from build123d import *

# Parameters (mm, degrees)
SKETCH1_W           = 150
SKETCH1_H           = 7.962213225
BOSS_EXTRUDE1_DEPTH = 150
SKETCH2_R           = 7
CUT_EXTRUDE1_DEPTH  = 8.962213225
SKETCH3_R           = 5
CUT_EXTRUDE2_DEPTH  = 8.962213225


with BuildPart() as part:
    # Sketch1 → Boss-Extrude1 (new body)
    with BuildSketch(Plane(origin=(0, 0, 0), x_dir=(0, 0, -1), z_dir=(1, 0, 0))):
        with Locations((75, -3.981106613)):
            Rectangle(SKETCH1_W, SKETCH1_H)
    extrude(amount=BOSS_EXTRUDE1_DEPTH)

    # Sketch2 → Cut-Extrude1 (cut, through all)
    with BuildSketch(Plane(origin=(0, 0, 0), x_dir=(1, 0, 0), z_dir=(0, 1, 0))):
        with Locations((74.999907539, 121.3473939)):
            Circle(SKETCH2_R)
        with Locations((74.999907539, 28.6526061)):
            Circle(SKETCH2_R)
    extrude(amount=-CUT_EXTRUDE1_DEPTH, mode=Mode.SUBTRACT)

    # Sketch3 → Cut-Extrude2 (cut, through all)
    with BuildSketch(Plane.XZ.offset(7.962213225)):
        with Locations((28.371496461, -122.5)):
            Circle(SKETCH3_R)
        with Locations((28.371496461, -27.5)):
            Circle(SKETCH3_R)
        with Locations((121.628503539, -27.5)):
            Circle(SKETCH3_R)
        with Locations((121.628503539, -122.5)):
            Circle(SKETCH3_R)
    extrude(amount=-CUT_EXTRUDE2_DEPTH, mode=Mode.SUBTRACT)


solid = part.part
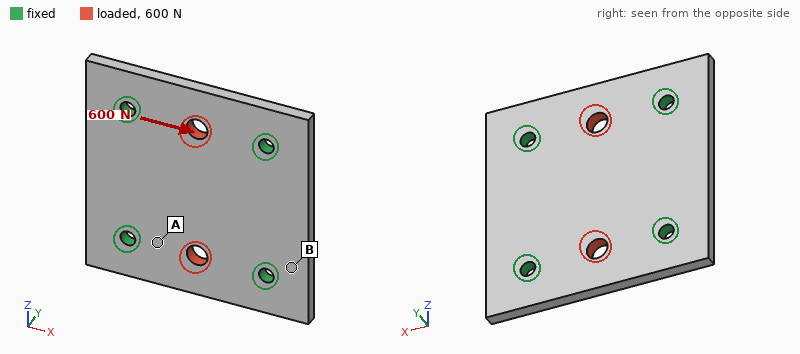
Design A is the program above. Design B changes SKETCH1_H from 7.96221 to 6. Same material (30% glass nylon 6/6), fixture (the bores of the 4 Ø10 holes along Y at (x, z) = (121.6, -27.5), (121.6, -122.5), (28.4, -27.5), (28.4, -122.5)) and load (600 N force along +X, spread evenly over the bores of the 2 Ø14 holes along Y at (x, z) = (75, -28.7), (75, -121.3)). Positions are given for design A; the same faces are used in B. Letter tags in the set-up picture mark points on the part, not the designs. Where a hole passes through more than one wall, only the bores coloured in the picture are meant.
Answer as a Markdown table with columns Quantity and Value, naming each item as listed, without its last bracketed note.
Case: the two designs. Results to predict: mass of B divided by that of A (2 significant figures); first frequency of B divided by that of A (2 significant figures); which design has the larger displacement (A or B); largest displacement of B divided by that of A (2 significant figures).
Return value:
| Quantity | Value |
|---|---|
| mass of B divided by that of A | 0.75 |
| first frequency of B divided by that of A | 0.78 |
| which design has the larger displacement | B |
| largest displacement of B divided by that of A | 1.3 |
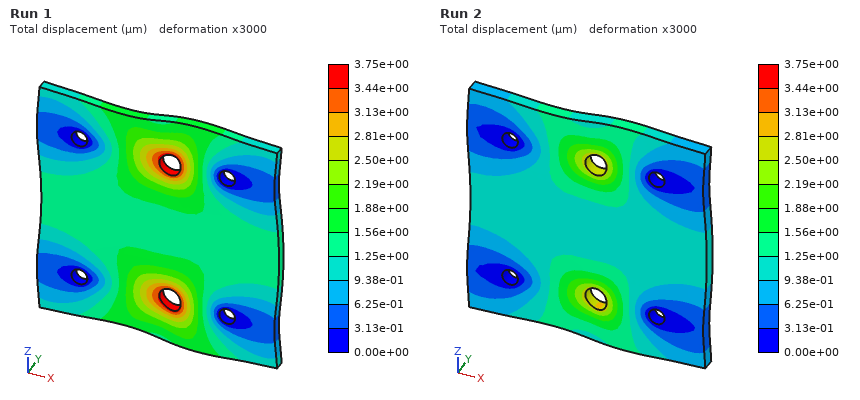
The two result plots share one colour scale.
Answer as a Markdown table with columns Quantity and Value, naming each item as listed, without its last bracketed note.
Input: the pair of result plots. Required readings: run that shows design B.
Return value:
| Quantity | Value |
|---|---|
| run that shows design B | Run 1 |
